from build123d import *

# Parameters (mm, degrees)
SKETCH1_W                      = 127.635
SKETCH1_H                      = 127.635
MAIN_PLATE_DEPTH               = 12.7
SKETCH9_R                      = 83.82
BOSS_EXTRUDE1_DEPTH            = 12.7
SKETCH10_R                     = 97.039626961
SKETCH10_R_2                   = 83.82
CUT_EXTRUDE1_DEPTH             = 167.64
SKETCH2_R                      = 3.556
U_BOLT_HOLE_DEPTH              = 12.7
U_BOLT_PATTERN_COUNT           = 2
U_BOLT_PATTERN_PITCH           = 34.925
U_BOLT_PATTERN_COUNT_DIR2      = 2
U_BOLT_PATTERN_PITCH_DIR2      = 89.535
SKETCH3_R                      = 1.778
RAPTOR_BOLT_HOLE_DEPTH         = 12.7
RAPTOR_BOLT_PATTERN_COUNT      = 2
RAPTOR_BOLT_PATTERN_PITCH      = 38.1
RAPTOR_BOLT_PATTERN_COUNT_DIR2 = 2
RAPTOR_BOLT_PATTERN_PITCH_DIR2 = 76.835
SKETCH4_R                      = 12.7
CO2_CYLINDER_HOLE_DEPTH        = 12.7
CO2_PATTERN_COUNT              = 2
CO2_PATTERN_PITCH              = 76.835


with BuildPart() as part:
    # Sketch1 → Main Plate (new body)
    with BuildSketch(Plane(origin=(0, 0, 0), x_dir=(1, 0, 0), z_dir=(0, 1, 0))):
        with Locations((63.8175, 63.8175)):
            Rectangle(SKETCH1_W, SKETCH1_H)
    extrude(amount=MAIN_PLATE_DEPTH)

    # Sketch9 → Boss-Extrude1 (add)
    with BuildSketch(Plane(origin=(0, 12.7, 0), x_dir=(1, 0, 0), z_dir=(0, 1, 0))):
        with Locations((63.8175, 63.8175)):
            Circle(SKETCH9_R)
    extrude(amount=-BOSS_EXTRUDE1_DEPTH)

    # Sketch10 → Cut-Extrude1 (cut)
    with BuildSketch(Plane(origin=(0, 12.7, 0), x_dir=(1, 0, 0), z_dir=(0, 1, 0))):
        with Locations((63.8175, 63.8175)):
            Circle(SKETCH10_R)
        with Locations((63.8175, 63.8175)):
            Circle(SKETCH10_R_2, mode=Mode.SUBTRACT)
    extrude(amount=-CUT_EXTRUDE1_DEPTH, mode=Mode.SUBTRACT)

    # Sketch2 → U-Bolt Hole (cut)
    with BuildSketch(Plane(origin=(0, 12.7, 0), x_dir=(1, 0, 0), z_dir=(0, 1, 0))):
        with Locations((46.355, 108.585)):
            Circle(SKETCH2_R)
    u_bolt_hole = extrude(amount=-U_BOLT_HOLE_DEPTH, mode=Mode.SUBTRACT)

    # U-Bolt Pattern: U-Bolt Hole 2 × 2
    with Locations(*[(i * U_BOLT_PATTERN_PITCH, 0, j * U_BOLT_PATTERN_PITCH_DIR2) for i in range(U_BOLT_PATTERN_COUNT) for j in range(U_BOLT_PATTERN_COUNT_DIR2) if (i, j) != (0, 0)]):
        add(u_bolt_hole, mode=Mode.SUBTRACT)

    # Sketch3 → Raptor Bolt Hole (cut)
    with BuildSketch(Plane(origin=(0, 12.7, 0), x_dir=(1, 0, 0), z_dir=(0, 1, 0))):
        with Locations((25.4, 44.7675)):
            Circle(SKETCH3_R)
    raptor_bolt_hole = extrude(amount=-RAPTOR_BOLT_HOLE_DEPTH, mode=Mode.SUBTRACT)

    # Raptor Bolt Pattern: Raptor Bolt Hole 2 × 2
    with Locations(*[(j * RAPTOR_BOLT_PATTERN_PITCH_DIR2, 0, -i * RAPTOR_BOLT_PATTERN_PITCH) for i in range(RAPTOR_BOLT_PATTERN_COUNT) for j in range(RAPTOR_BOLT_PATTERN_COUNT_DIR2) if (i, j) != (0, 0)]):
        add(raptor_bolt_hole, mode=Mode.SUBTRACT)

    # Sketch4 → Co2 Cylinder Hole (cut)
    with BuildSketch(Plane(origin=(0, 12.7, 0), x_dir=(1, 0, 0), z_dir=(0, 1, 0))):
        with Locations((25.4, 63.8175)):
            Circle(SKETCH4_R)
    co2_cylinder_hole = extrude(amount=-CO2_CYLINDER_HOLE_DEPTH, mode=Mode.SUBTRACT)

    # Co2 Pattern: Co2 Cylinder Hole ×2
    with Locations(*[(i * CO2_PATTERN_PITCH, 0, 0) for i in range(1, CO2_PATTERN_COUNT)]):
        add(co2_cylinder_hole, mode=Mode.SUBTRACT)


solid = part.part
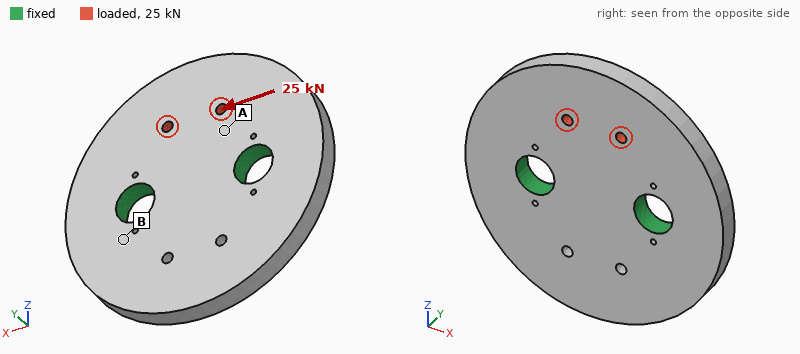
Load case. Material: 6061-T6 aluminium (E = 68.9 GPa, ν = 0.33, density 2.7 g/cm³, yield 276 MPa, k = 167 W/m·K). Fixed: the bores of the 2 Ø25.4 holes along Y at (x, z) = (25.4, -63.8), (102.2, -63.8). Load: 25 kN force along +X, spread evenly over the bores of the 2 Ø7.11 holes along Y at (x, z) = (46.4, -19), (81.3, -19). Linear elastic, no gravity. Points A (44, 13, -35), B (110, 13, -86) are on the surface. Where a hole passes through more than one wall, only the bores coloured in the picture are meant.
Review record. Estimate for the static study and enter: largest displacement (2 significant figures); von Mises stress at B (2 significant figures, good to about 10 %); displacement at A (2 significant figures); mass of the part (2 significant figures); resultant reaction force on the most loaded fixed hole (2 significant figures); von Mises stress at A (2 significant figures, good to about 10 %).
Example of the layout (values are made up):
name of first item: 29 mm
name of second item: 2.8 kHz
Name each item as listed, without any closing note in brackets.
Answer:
largest displacement: 34 µm
von Mises stress at B: 6.5 MPa
displacement at A: 16 µm
mass of the part: 720 g
resultant reaction force on the most loaded fixed hole: 16 kN
von Mises stress at A: 34 MPa
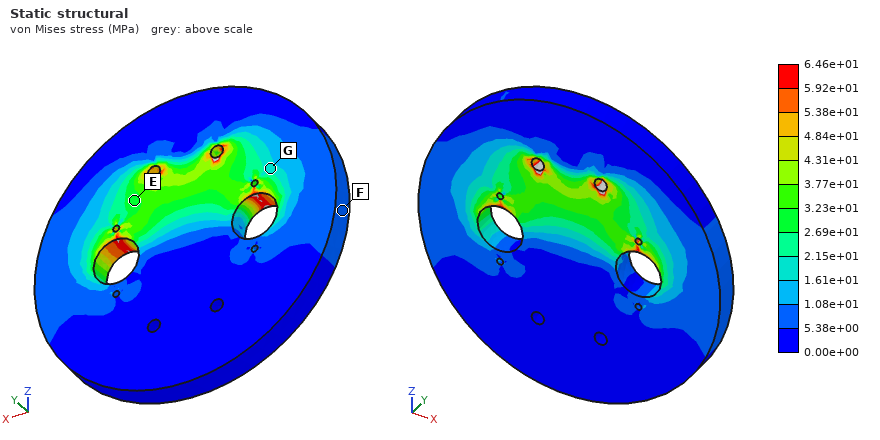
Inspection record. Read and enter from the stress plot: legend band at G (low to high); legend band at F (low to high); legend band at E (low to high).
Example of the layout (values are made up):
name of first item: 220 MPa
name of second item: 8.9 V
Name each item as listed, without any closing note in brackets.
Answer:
legend band at G: 1.61e+01 to 2.15e+01 MPa
legend band at F: 5.38e+00 to 1.08e+01 MPa
legend band at E: 2.69e+01 to 3.23e+01 MPa
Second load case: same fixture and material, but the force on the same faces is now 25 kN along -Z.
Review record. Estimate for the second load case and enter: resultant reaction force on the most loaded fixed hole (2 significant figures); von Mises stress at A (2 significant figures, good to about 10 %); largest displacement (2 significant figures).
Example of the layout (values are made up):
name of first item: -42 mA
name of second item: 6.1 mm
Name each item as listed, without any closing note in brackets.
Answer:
resultant reaction force on the most loaded fixed hole: 13 kN
von Mises stress at A: 29 MPa
largest displacement: 20 µm
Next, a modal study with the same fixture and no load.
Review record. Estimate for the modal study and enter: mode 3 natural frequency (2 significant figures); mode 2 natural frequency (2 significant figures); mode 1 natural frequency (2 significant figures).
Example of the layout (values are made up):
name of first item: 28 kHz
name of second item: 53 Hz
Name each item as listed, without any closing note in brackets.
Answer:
mode 3 natural frequency: 4000 Hz
mode 2 natural frequency: 2300 Hz
mode 1 natural frequency: 2200 Hz
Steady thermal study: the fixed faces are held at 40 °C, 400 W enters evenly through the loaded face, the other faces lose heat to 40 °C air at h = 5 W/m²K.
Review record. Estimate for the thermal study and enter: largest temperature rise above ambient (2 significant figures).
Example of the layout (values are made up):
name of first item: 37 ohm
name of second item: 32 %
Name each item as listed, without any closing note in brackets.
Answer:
largest temperature rise above ambient: 84 K
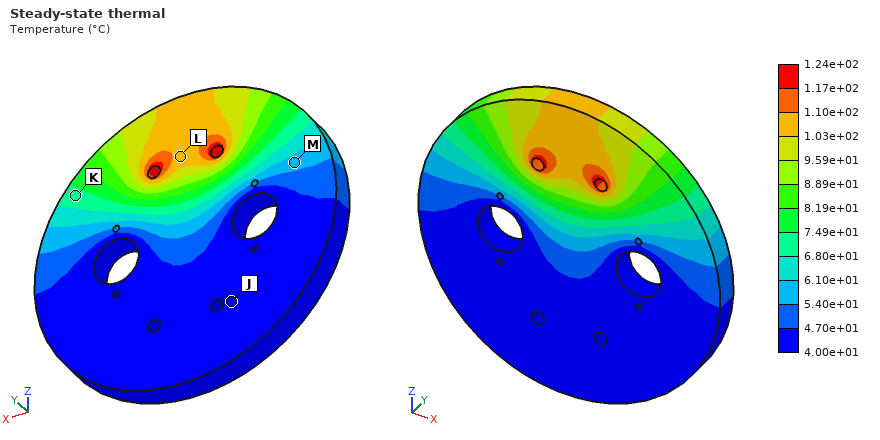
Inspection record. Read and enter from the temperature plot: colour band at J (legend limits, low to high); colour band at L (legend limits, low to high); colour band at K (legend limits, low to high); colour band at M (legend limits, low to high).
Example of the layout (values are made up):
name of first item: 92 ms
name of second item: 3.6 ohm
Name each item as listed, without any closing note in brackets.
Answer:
colour band at J: 4.00e+01 to 4.70e+01 °C
colour band at L: 1.03e+02 to 1.10e+02 °C
colour band at K: 6.80e+01 to 7.49e+01 °C
colour band at M: 5.40e+01 to 6.10e+01 °C
